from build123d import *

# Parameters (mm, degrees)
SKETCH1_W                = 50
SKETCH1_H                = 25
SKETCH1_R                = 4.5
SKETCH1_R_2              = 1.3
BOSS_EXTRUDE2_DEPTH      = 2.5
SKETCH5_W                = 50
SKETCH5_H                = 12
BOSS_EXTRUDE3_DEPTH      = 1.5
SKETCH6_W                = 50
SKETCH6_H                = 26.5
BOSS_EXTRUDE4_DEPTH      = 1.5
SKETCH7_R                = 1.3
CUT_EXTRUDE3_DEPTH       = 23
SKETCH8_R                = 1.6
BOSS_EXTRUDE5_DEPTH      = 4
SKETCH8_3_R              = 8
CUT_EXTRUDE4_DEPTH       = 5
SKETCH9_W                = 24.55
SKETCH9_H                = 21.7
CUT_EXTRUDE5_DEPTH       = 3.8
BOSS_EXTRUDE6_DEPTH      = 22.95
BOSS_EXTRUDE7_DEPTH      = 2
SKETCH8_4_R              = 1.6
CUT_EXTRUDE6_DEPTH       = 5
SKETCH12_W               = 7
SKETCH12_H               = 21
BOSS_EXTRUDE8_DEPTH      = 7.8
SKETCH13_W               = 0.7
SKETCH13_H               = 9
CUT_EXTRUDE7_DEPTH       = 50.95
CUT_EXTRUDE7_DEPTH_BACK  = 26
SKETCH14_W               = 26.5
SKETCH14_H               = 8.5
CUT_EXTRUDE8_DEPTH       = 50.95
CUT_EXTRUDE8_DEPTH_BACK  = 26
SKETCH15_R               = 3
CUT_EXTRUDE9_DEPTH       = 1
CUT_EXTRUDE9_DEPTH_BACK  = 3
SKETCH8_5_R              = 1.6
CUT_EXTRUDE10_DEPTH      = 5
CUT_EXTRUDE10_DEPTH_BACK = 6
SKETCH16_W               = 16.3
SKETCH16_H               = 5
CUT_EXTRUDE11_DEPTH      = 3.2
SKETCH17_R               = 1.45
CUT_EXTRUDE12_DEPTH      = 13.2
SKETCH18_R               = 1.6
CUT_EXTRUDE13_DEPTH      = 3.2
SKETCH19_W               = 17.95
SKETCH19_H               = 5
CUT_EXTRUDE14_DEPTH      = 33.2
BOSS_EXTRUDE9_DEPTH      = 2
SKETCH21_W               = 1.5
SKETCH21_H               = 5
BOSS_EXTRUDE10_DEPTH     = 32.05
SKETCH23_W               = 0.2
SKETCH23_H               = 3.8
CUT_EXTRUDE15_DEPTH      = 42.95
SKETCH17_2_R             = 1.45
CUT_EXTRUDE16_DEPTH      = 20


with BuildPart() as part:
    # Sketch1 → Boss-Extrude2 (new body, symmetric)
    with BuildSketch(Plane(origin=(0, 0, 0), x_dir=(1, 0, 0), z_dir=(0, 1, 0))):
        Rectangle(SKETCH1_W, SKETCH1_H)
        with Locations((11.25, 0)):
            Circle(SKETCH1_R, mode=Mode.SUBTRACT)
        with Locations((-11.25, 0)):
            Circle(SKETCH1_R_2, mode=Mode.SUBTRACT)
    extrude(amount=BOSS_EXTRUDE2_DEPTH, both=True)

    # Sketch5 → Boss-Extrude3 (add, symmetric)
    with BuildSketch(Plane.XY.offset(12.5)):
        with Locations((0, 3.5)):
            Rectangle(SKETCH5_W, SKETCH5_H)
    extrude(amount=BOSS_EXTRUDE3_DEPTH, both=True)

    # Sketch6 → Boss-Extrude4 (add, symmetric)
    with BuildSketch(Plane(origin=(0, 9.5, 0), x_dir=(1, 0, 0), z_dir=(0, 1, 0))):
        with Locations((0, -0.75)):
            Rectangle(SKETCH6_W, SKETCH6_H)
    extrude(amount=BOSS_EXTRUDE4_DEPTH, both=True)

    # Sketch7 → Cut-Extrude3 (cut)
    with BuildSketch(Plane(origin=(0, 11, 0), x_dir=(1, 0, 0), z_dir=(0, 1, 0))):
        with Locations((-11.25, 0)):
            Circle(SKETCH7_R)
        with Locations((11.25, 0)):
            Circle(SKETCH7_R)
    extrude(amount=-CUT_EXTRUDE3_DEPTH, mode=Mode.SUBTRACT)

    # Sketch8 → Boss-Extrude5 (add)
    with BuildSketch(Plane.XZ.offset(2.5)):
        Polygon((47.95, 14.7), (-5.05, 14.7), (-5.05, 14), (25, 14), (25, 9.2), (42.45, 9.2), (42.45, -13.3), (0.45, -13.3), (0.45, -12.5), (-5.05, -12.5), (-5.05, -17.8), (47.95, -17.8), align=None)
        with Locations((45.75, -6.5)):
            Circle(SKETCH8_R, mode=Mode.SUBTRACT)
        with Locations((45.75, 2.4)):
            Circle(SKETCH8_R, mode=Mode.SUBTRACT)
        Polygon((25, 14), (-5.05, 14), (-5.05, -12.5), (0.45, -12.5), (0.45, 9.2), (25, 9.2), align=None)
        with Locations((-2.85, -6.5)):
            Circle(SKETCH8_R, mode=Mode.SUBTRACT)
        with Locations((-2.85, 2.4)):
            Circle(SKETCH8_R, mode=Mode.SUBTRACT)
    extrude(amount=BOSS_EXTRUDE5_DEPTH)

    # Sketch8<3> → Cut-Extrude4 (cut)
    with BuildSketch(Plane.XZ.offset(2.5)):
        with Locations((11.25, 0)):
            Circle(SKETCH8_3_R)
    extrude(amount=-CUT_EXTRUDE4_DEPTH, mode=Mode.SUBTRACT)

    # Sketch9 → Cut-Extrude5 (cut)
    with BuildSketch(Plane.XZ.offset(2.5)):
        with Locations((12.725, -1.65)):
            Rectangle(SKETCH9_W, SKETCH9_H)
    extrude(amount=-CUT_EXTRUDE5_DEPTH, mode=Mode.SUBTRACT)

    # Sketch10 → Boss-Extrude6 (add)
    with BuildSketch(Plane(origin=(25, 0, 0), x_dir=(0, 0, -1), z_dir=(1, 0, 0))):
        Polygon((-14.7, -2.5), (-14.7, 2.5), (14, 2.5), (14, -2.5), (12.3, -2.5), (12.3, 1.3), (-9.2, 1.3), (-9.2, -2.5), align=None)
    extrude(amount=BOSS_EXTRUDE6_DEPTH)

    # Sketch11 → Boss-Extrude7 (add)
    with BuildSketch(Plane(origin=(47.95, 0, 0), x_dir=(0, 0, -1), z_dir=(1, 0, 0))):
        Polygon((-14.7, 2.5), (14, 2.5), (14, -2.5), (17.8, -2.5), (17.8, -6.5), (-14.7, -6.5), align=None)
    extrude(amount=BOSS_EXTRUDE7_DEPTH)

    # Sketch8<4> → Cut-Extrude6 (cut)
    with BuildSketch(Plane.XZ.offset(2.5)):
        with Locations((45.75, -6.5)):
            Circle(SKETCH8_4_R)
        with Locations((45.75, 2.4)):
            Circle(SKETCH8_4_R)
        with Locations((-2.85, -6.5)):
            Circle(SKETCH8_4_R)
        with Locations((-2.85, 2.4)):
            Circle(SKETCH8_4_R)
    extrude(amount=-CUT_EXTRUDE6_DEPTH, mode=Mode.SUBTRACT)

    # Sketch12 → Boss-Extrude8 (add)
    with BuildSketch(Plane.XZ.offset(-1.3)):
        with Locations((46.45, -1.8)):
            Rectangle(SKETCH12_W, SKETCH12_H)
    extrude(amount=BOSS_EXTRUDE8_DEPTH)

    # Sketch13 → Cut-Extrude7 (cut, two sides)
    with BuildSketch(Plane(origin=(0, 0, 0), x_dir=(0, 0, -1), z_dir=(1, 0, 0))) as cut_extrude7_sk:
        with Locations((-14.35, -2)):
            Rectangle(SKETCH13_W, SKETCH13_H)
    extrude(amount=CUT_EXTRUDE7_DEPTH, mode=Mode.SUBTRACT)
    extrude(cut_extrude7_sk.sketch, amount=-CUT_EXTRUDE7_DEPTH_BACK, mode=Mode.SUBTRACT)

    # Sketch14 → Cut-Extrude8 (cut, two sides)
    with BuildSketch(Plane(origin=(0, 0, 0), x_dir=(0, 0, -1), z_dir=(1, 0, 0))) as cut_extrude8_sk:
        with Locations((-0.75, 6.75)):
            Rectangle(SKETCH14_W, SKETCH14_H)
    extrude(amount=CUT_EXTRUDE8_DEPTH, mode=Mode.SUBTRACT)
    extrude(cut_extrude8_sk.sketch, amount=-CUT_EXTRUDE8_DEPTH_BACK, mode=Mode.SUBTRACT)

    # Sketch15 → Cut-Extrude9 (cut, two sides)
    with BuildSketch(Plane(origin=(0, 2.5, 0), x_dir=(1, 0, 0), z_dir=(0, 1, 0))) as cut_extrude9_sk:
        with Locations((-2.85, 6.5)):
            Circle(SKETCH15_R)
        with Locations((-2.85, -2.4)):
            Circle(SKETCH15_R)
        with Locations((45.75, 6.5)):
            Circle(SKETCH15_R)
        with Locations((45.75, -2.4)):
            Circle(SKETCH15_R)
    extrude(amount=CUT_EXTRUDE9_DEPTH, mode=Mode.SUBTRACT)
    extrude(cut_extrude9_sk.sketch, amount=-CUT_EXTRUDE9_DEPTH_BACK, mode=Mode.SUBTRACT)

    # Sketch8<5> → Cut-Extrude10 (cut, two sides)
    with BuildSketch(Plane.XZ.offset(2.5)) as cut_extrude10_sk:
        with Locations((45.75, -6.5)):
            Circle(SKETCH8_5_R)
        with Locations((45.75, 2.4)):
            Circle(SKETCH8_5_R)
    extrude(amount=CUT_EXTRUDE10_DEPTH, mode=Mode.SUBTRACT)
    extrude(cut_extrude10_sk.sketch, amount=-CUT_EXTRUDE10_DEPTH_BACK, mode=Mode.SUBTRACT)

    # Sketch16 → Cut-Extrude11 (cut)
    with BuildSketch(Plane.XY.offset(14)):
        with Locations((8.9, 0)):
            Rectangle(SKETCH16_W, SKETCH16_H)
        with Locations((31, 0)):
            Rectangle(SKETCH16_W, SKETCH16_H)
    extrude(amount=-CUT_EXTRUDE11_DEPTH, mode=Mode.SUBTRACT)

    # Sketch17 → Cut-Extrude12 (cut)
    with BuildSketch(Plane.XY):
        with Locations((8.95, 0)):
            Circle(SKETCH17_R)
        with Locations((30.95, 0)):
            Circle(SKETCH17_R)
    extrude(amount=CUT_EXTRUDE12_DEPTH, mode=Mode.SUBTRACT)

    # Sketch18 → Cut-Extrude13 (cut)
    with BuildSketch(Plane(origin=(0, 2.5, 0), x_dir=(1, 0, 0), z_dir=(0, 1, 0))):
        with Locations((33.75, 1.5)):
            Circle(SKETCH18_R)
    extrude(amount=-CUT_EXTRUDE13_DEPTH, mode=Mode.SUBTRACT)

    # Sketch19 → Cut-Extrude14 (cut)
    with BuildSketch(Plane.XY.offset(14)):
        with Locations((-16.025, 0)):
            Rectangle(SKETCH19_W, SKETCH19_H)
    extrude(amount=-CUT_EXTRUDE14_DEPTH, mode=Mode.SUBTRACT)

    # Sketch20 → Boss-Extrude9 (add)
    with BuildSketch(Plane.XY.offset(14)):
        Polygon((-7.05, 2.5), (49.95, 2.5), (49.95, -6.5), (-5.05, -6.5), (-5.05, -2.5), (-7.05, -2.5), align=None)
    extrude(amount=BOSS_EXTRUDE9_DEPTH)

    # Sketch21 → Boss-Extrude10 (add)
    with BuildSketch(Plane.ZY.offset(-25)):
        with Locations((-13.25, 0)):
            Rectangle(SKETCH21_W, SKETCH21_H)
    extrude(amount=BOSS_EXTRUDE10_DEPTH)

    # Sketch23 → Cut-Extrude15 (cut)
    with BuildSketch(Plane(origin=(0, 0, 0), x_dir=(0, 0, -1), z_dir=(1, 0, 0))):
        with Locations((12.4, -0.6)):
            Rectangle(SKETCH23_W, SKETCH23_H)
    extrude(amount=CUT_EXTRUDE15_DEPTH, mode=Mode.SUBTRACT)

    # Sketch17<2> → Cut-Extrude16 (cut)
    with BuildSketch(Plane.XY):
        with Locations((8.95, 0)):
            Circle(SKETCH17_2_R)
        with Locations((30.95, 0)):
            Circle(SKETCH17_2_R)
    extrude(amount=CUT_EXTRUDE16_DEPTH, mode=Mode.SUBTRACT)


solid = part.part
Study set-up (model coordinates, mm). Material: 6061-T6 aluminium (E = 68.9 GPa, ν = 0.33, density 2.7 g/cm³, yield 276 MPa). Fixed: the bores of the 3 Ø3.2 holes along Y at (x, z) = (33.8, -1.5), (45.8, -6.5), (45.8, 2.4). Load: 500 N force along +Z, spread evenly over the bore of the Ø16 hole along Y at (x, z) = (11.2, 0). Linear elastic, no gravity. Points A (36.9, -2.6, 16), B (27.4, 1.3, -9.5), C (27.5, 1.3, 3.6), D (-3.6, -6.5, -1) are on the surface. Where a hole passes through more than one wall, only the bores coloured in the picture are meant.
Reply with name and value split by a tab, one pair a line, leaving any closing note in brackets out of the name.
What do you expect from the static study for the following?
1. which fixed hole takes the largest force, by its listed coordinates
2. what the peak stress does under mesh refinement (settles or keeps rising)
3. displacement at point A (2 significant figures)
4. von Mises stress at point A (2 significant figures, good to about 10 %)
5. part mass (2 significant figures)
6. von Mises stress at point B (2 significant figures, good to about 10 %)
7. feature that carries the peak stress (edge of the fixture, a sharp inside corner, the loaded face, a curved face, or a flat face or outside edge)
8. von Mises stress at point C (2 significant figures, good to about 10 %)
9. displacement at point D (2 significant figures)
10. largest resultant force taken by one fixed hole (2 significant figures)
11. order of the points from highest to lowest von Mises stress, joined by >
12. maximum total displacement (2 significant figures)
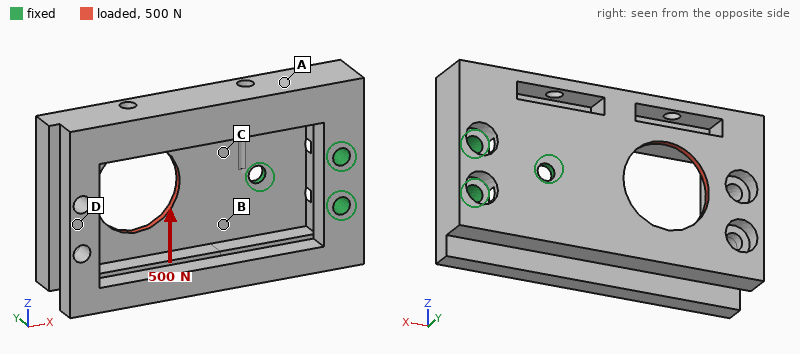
which fixed hole takes the largest force, by its listed coordinates	(33.8, -1.5)
what the peak stress does under mesh refinement	keeps rising
displacement at point A	16 µm
von Mises stress at point A	15 MPa
part mass	20 g
von Mises stress at point B	27 MPa
feature that carries the peak stress	edge of the fixture
von Mises stress at point C	40 MPa
displacement at point D	73 µm
largest resultant force taken by one fixed hole	760 N
order of the points from highest to lowest von Mises stress, joined by >	C > B > A > D
maximum total displacement	82 µm
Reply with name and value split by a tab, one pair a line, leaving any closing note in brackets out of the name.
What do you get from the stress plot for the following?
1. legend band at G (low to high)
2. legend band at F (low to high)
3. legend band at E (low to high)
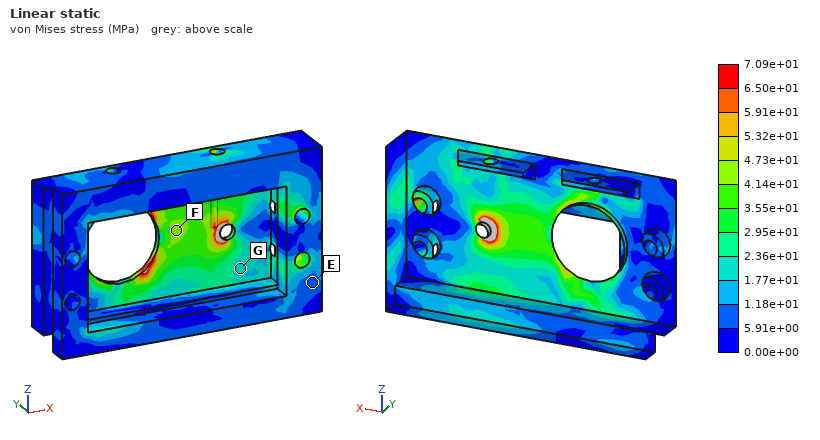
legend band at G	1.77e+01 to 2.36e+01 MPa
legend band at F	4.14e+01 to 4.73e+01 MPa
legend band at E	5.91e+00 to 1.18e+01 MPa
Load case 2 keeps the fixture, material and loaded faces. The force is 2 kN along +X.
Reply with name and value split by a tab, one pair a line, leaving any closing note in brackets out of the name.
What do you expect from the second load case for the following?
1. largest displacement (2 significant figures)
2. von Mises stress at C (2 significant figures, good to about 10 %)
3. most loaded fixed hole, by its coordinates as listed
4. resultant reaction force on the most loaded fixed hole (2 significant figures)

largest displacement	0.15 mm
von Mises stress at C	57 MPa
most loaded fixed hole, by its coordinates as listed	(33.8, -1.5)
resultant reaction force on the most loaded fixed hole	1.3 kN
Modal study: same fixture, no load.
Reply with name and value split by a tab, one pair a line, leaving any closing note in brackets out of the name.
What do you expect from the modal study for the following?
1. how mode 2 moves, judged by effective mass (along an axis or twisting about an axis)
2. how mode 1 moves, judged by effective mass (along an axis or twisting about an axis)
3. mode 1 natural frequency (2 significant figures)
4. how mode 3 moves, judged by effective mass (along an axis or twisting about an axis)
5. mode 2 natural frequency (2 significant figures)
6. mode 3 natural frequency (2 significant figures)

how mode 2 moves, judged by effective mass	along Z
how mode 1 moves, judged by effective mass	along Y
mode 1 natural frequency	1900 Hz
how mode 3 moves, judged by effective mass	along Z
mode 2 natural frequency	2800 Hz
mode 3 natural frequency	4800 Hz
